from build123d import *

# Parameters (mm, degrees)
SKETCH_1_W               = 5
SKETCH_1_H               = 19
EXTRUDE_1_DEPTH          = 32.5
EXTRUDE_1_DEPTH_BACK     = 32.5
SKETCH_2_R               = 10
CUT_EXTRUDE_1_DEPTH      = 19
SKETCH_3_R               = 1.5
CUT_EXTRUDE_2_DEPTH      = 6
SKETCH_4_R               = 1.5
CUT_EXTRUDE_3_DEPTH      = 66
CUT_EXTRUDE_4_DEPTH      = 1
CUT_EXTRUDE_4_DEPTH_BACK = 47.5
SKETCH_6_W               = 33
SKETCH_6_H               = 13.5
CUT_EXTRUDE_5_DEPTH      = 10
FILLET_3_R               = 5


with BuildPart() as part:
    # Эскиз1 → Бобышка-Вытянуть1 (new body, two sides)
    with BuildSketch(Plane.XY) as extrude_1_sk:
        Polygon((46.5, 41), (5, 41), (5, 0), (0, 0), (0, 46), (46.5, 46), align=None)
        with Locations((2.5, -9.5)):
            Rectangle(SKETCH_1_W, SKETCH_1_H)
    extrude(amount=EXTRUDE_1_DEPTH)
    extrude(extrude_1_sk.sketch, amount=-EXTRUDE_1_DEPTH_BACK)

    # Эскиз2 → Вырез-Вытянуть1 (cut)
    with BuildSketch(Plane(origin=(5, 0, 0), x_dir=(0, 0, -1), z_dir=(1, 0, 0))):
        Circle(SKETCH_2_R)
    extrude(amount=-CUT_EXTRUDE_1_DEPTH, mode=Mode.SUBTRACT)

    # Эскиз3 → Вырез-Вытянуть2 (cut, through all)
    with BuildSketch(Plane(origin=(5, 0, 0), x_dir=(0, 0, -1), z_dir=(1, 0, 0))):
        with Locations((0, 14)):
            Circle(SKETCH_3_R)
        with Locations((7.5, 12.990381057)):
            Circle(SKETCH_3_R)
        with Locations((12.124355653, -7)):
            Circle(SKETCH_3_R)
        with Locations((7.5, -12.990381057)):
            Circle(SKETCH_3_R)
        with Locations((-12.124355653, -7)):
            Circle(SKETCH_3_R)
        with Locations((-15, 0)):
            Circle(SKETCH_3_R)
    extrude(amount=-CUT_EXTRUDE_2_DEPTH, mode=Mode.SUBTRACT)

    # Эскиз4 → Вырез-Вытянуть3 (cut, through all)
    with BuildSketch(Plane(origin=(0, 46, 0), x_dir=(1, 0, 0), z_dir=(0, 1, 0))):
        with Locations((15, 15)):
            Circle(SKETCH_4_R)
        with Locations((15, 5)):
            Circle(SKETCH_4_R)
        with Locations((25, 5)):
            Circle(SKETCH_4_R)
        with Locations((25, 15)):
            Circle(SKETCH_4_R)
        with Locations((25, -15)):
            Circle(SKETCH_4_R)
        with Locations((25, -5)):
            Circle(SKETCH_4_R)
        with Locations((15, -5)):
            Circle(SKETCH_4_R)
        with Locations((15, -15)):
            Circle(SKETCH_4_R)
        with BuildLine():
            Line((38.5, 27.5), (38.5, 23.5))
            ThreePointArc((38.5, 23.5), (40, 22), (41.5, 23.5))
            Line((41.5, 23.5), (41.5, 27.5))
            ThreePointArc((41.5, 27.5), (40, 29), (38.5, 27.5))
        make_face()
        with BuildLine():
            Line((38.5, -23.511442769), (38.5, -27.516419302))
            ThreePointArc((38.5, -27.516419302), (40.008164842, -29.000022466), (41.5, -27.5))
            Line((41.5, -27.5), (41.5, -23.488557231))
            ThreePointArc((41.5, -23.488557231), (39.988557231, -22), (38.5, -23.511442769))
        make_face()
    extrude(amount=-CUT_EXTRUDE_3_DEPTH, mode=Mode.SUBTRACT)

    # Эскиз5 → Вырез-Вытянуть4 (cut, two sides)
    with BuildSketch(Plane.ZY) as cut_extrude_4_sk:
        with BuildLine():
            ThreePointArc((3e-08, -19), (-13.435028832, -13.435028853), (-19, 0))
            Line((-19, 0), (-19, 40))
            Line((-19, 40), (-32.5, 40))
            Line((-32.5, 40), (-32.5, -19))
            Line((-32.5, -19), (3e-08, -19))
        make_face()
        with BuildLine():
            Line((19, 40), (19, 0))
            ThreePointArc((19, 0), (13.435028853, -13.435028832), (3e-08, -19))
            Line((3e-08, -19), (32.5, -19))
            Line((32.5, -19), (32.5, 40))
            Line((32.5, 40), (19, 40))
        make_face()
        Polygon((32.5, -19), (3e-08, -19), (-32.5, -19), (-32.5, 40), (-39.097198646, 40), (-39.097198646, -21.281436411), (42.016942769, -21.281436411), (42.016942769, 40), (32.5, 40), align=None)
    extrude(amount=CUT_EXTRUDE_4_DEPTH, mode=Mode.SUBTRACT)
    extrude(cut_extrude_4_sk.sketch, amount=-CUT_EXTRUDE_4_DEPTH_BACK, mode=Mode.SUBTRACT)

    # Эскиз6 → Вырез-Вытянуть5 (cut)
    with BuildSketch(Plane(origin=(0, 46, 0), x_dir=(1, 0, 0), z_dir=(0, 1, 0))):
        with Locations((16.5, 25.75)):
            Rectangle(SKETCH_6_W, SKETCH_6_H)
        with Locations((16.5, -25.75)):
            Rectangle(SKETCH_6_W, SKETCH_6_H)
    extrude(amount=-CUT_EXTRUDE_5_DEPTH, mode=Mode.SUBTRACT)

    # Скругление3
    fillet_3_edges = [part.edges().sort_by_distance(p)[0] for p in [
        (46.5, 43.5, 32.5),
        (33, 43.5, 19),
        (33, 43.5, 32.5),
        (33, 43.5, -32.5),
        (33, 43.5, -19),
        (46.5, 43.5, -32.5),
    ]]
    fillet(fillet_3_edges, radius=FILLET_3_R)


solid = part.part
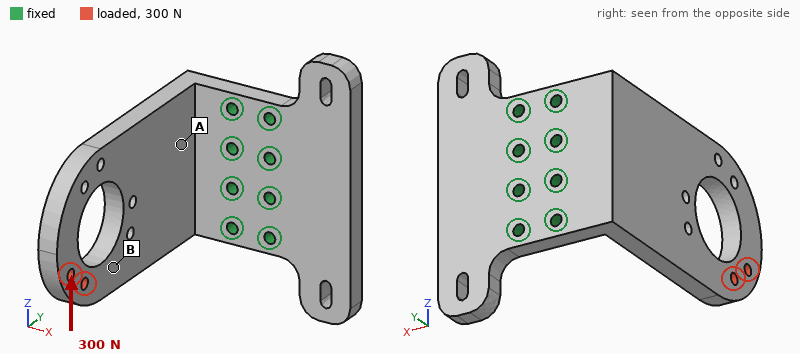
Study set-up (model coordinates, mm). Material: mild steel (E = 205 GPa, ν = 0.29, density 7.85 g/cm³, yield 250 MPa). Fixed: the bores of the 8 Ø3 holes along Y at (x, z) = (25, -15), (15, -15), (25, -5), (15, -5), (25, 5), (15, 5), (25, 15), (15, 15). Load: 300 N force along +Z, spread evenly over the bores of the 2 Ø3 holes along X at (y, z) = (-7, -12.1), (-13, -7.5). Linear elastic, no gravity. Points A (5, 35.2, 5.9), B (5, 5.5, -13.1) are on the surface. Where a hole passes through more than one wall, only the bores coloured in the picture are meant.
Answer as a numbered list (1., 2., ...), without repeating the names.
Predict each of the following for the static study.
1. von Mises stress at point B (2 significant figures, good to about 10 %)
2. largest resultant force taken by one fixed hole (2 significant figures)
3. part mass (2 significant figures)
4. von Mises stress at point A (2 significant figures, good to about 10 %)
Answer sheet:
1. 8.1 MPa
2. 500 N
3. 150 g
4. 17 MPa
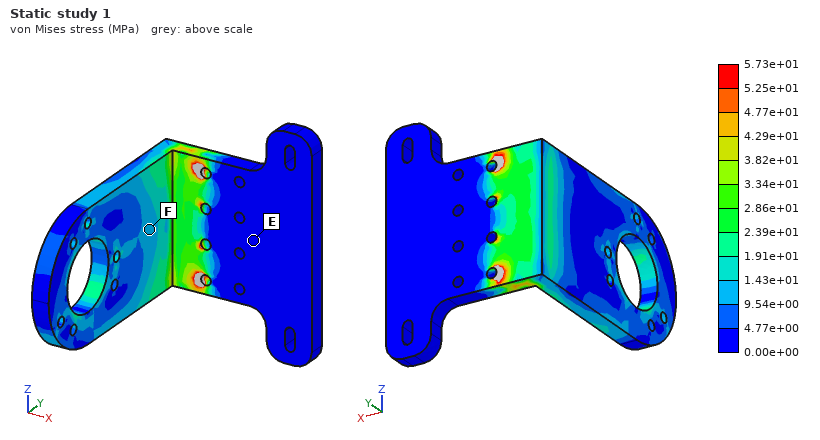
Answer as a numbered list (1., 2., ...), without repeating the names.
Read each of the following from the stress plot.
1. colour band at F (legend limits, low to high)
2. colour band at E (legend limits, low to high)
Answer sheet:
1. 9.54e+00 to 1.43e+01 MPa
2. 0.00e+00 to 4.77e+00 MPa
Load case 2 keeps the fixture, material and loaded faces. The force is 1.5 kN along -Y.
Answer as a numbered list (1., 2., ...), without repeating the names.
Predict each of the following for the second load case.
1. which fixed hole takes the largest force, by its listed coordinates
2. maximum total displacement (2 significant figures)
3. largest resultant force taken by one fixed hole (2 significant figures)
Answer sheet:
1. (15, -15)
2. 93 µm
3. 860 N
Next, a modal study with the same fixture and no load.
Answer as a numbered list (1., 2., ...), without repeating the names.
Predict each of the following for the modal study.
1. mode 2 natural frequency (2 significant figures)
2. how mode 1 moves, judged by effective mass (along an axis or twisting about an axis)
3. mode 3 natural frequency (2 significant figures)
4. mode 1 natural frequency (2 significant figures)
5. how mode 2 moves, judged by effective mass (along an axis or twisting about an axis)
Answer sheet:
1. 3000 Hz
2. along X
3. 4200 Hz
4. 1100 Hz
5. along Z
